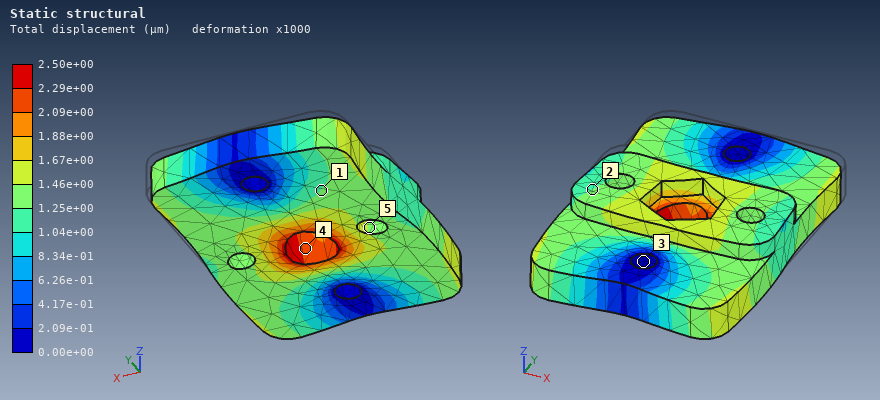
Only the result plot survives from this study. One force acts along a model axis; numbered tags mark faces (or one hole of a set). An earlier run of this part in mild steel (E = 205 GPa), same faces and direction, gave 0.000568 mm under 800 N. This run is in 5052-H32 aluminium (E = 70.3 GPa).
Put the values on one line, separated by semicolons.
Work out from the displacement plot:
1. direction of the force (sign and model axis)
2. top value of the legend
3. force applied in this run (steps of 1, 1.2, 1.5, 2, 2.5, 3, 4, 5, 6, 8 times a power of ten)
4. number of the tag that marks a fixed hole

-Y; 2.50e+00 µm; 1.2 kN; 3
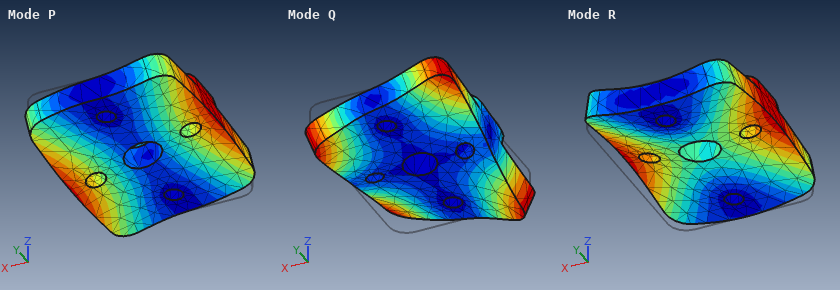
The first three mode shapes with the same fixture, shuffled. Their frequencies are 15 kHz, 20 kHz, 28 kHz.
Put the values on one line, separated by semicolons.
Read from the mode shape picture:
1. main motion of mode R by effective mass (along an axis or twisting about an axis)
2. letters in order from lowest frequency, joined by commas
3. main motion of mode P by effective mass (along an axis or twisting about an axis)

along Z; P, R, Q; twisting about Y
